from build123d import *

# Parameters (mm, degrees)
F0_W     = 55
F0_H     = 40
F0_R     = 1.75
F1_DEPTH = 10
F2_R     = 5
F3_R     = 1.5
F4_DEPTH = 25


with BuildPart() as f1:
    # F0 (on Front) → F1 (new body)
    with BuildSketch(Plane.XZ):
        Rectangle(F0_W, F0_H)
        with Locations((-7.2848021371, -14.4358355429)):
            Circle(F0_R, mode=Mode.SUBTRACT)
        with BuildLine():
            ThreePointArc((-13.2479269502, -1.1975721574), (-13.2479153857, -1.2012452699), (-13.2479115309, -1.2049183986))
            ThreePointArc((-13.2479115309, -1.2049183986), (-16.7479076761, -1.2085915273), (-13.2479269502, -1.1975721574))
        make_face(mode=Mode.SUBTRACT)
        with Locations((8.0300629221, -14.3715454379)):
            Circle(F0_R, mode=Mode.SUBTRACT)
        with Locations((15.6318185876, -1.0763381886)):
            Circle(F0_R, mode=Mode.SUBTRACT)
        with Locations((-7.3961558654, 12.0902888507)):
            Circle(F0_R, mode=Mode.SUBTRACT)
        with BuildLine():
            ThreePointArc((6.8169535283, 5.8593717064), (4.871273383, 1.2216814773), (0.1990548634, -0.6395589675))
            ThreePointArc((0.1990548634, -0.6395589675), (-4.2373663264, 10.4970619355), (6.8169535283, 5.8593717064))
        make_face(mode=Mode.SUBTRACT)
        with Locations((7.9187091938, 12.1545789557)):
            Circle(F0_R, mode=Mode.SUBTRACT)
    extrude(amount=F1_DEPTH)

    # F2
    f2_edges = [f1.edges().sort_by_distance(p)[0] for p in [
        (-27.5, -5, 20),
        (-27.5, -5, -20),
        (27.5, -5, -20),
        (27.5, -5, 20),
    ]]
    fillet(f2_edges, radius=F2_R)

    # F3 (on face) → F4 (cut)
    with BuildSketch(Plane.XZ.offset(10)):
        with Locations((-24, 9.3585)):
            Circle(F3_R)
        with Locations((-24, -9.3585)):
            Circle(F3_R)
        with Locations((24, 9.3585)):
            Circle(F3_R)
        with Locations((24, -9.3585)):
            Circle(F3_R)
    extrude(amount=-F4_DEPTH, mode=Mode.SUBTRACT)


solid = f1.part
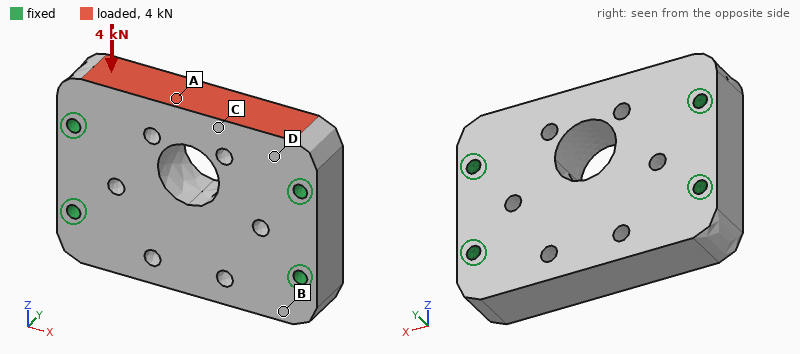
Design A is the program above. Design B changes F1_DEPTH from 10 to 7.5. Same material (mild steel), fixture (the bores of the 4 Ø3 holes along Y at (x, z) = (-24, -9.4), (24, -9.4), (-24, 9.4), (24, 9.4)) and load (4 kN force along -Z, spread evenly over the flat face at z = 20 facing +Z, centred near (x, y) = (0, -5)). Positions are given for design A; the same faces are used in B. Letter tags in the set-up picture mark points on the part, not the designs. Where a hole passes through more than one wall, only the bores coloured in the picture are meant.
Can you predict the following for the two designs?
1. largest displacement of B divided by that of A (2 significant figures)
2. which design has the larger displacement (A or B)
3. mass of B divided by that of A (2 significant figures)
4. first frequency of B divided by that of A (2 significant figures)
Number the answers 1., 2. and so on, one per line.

1. 1.3
2. B
3. 0.75
4. 0.83
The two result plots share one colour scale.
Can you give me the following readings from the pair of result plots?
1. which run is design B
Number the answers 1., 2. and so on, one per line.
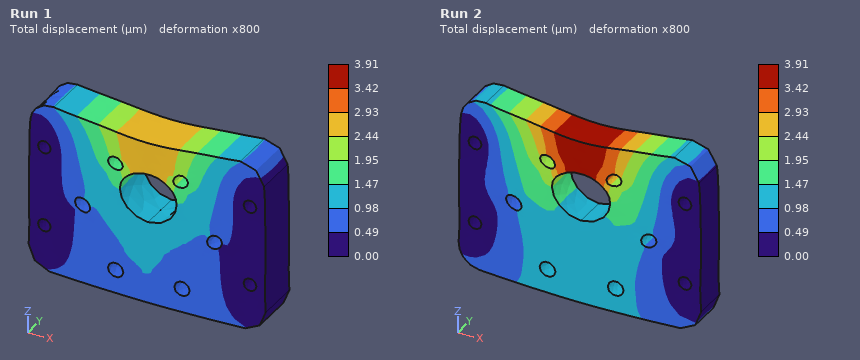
1. Run 2
